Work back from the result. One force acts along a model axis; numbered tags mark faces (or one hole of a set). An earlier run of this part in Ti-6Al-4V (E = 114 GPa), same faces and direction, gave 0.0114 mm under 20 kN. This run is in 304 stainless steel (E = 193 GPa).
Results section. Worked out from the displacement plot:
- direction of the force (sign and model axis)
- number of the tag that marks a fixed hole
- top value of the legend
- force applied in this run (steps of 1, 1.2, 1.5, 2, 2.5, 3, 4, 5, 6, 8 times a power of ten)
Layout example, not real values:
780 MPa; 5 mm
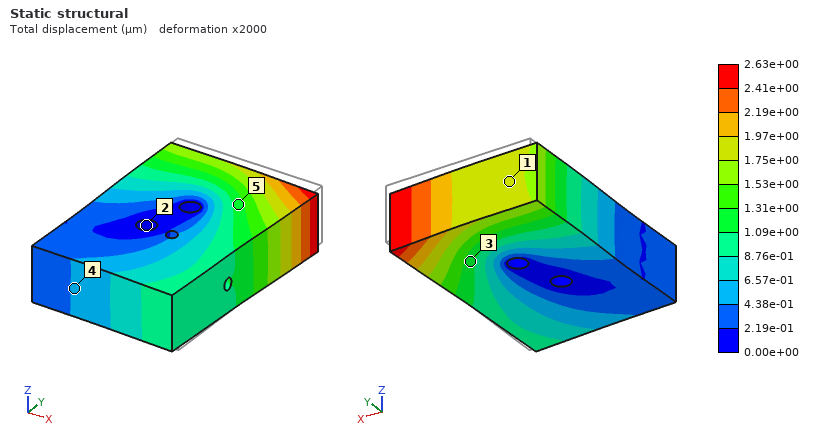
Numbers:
-Y; 2; 2.63e+00 µm; 8 kN
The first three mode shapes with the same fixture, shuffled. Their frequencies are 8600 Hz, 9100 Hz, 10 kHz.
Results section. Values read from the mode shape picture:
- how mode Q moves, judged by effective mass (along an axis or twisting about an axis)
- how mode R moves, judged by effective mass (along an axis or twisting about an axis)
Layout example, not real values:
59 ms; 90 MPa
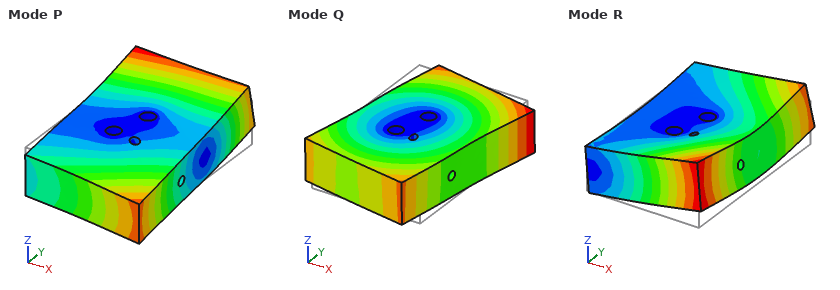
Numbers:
twisting about Z; along Z
